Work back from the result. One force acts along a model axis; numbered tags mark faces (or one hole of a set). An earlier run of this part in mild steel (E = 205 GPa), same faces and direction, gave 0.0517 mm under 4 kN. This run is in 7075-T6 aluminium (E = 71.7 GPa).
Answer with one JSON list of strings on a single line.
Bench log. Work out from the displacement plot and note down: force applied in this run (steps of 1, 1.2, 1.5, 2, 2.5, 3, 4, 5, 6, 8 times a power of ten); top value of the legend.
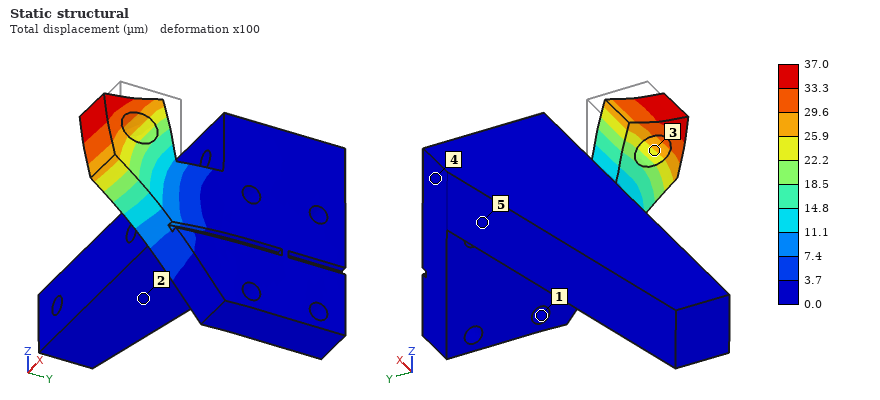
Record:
["1 kN", "37.0 µm"]
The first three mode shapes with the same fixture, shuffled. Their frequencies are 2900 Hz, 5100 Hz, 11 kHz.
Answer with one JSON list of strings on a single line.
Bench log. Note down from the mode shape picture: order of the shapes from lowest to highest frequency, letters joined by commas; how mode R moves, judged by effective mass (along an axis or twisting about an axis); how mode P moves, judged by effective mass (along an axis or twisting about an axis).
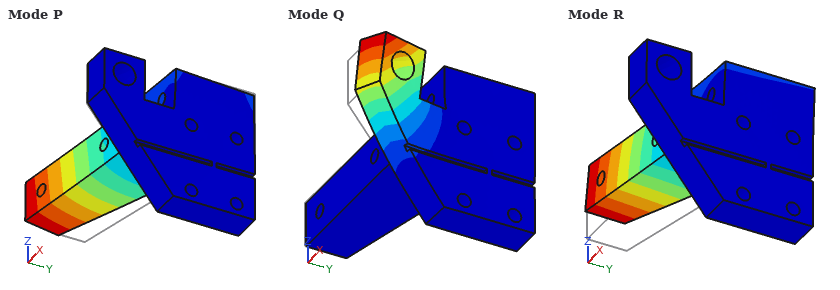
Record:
["R, P, Q", "along Z", "along Y"]
